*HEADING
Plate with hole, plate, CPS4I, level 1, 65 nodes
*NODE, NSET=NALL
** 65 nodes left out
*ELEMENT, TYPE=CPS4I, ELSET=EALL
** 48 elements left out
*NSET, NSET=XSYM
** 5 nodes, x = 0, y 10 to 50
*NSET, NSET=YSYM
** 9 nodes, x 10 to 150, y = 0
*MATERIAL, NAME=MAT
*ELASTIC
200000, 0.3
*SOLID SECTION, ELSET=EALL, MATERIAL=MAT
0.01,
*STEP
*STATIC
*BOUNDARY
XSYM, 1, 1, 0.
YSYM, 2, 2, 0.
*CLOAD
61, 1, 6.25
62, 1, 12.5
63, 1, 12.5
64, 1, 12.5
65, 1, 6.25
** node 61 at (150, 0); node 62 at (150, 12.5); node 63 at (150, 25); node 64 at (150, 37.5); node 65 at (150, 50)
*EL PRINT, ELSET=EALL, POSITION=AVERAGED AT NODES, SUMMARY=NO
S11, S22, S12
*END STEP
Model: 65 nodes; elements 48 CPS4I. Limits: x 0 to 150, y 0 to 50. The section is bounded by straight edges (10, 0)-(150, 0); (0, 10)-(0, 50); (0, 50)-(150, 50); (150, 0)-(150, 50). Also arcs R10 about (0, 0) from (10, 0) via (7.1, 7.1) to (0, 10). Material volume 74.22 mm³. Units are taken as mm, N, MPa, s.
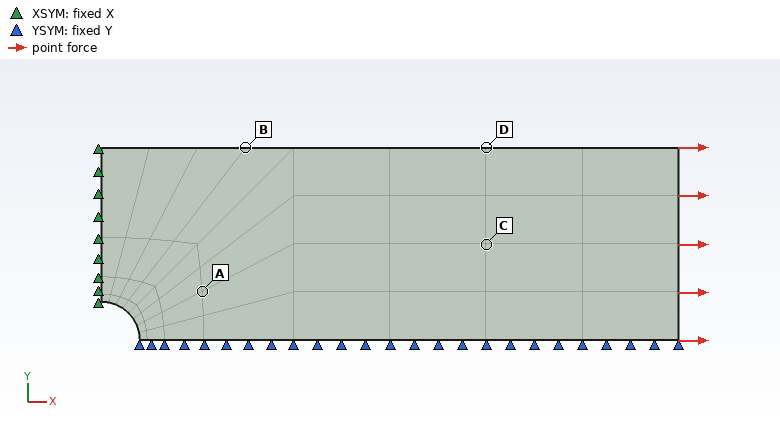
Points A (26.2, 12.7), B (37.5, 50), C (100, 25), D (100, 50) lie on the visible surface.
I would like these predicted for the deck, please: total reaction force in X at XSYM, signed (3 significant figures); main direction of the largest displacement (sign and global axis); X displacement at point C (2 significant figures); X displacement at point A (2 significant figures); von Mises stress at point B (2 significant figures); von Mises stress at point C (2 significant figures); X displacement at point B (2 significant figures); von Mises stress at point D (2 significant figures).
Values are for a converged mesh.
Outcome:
-50.0 N
+X
0.052 mm
0.017 mm
110 MPa
99 MPa
0.020 mm
100 MPa
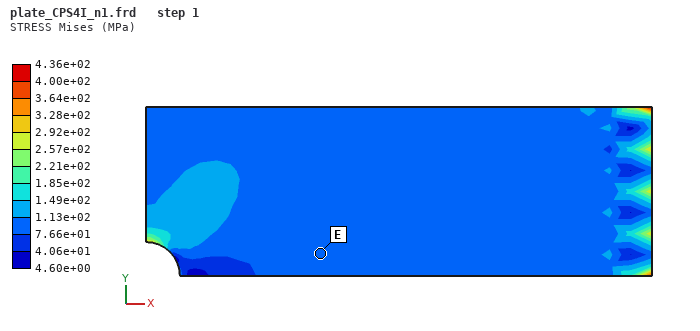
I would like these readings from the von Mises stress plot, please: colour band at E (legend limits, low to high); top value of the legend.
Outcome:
7.66e+01 to 1.13e+02 MPa
4.36e+02 MPa
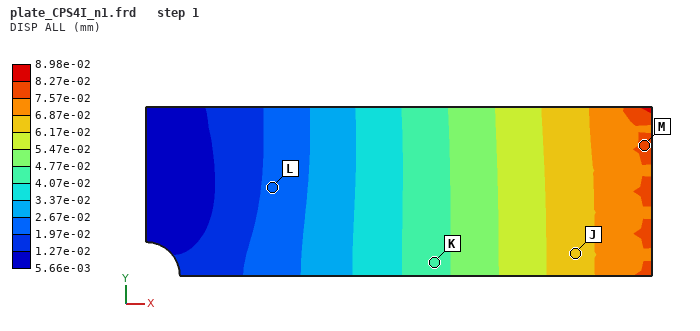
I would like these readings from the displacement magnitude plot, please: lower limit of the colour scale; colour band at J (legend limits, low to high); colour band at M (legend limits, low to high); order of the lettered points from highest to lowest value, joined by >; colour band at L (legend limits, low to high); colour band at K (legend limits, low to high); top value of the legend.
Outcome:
5.66e-03 mm
6.17e-02 to 6.87e-02 mm
7.57e-02 to 8.27e-02 mm
M > J > K > L
1.97e-02 to 2.67e-02 mm
4.07e-02 to 4.77e-02 mm
8.98e-02 mm
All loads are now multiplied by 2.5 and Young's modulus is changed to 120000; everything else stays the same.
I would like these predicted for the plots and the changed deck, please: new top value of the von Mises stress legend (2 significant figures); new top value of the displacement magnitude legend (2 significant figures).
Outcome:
1100 MPa
0.37 mm
